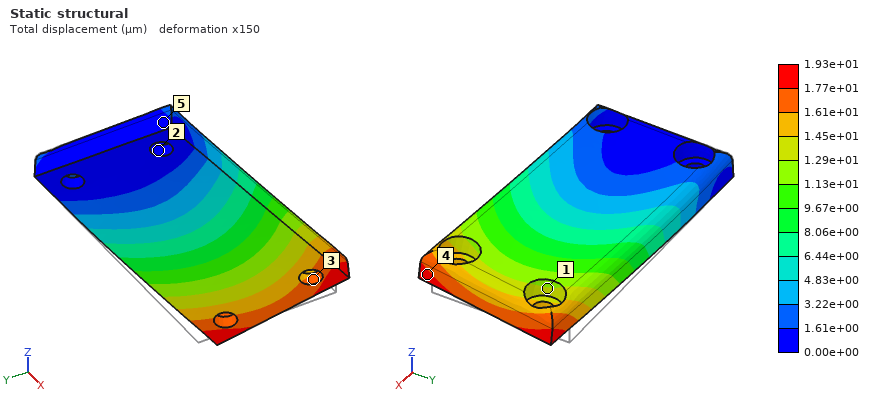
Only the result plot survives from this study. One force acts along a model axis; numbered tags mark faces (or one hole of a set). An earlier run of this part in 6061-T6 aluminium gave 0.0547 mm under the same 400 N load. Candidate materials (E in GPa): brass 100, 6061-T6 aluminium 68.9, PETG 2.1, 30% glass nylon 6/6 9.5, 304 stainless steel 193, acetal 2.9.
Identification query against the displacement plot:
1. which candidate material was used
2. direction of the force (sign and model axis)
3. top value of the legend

304 stainless steel
-Y
1.93e+01 µm
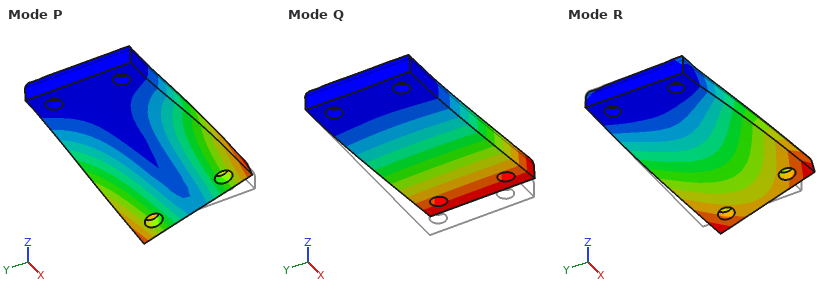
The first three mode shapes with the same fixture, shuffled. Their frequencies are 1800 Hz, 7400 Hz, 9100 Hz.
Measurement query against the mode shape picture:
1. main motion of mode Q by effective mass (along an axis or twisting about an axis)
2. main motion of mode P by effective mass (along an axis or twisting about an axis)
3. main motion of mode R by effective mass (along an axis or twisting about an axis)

along Z
along Y
along Y
